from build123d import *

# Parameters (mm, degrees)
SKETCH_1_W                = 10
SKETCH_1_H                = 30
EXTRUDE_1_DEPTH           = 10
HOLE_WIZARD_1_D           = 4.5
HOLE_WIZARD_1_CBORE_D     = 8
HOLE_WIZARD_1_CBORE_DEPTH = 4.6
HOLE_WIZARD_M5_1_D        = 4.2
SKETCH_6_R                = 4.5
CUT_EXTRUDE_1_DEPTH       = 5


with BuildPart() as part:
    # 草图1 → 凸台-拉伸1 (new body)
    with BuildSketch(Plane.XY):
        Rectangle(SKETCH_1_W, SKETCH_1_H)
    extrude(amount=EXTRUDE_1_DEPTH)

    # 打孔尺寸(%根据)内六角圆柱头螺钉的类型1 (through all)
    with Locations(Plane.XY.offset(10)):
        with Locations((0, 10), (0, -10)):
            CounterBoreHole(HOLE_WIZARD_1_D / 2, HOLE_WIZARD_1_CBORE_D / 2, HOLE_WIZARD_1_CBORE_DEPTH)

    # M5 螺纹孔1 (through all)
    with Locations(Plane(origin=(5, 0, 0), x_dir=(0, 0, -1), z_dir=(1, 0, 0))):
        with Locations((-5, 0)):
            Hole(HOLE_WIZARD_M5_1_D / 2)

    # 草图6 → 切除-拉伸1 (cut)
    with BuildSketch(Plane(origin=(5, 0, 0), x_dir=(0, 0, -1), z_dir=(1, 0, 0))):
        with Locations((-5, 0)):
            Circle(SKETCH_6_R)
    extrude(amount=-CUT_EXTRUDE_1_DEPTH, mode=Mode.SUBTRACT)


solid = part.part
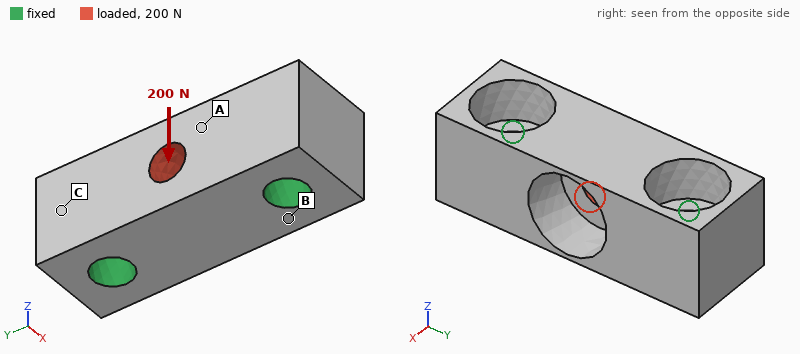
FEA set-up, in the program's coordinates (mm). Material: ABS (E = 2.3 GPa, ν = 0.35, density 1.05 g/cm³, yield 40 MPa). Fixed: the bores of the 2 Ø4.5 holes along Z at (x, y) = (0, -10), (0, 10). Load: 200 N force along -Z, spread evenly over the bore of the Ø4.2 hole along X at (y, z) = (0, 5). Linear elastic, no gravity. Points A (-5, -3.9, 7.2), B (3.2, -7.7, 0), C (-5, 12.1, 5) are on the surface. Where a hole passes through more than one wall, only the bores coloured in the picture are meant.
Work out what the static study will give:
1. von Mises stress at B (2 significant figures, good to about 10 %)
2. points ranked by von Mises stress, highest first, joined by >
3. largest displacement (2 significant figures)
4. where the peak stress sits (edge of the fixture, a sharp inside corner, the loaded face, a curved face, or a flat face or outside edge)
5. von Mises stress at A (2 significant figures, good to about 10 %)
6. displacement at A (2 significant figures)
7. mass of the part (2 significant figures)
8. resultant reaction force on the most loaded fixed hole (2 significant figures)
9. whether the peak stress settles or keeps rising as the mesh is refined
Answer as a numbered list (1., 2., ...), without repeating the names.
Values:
1. 2.1 MPa
2. A > B > C
3. 40 µm
4. edge of the fixture
5. 3.9 MPa
6. 29 µm
7. 2.1 g
8. 100 N
9. keeps rising
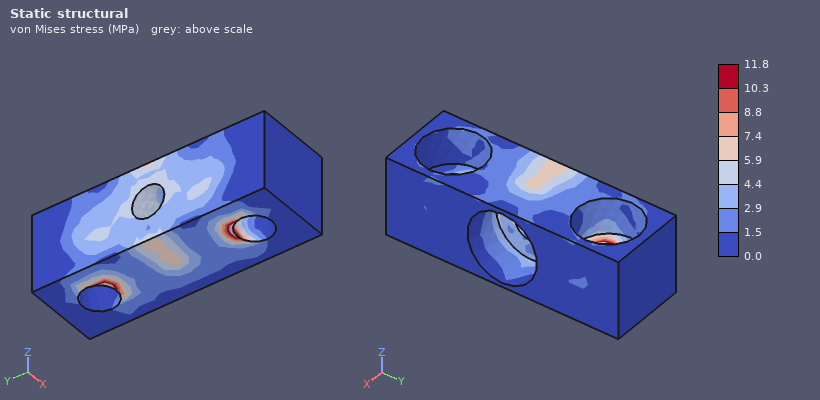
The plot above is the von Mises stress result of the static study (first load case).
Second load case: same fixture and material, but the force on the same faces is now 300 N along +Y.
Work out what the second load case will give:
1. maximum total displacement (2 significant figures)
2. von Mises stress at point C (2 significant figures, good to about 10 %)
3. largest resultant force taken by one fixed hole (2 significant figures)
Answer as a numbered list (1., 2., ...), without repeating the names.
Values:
1. 23 µm
2. 1.7 MPa
3. 150 N
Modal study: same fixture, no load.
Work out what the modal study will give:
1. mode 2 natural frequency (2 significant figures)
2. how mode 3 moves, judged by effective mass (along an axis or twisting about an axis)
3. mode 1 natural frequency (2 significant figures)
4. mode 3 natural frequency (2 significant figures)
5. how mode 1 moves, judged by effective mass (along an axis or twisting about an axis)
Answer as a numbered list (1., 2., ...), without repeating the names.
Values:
1. 18 kHz
2. along Z
3. 13 kHz
4. 19 kHz
5. along X
